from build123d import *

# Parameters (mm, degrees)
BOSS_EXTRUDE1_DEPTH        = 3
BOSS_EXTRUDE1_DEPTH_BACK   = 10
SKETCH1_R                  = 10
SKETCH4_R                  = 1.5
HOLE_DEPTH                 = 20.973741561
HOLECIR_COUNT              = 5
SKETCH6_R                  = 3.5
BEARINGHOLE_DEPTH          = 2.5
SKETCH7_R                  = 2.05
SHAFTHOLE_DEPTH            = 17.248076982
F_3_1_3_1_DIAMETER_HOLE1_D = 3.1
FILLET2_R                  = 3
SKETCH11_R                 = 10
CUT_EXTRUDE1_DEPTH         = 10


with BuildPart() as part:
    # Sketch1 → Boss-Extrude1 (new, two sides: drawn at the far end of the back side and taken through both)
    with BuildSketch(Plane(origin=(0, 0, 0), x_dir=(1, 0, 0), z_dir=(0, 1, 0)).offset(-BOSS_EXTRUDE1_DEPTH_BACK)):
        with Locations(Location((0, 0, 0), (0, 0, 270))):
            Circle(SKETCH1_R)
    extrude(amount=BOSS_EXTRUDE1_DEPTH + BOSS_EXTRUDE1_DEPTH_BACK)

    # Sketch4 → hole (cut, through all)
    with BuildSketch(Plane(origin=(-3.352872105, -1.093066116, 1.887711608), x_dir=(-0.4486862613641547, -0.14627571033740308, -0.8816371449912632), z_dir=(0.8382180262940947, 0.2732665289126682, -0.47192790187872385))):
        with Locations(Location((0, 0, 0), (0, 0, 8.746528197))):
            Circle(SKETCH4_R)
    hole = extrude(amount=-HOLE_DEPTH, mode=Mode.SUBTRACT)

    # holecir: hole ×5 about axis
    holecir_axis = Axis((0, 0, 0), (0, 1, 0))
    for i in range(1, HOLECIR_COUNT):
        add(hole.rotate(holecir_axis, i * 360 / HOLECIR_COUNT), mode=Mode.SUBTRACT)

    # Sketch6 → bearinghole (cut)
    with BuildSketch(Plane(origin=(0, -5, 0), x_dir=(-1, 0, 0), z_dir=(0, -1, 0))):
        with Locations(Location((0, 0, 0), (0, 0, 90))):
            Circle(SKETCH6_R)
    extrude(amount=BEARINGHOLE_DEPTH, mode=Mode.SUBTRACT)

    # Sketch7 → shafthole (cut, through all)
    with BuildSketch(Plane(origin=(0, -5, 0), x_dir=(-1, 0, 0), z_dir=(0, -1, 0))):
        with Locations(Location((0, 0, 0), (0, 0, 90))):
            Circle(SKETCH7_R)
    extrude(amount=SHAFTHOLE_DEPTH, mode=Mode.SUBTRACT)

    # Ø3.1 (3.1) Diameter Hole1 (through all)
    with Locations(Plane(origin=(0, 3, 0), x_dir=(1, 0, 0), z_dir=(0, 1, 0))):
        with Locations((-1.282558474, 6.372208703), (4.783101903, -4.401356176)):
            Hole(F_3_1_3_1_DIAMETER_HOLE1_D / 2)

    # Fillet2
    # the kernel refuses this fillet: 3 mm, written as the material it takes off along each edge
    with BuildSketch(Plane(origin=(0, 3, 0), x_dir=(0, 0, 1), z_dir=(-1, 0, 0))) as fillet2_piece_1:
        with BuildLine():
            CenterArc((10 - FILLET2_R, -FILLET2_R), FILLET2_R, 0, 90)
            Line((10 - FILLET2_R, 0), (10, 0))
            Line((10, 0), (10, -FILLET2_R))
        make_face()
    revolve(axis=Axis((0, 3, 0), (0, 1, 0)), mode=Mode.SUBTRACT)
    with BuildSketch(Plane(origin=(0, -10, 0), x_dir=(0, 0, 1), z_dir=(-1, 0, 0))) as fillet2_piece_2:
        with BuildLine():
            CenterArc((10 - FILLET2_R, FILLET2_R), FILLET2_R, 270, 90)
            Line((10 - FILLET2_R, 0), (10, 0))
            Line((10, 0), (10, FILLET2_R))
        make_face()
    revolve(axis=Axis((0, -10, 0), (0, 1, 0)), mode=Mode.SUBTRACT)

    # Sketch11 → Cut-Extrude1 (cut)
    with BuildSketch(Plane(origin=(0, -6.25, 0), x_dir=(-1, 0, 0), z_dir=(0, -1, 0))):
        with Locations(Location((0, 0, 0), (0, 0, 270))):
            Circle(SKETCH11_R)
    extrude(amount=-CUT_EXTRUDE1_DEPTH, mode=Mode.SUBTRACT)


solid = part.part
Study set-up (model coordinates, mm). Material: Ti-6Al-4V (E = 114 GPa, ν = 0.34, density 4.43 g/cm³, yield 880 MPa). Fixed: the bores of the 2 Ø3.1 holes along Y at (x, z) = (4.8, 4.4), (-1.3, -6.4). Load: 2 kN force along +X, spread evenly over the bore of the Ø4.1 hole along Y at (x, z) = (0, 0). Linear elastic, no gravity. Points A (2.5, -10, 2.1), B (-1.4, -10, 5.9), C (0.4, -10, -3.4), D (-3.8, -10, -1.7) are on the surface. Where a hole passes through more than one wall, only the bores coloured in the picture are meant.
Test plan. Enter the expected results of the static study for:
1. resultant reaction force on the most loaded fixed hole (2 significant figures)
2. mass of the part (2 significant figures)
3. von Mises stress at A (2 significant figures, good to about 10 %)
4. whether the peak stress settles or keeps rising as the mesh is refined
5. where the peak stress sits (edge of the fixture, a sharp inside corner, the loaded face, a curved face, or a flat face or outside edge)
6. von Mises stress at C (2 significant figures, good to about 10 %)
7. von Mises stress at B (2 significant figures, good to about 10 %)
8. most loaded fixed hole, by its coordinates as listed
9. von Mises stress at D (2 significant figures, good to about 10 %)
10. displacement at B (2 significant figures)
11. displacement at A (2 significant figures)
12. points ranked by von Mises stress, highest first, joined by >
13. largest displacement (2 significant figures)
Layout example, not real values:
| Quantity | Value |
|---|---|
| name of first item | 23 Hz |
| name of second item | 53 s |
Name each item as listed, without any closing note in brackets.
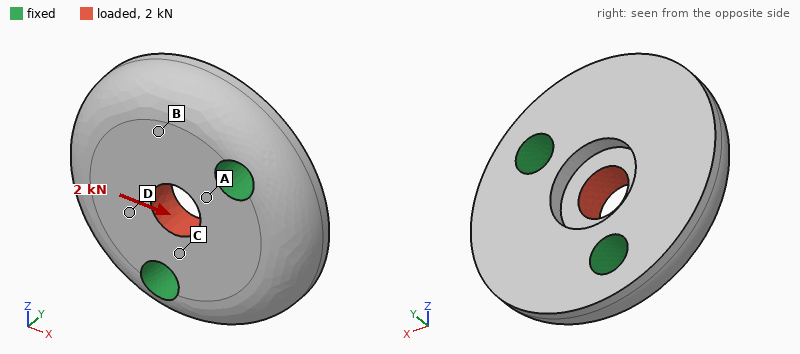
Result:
| Quantity | Value |
|---|---|
| resultant reaction force on the most loaded fixed hole | 1.1 kN |
| mass of the part | 4.1 g |
| von Mises stress at A | 67 MPa |
| whether the peak stress settles or keeps rising as the mesh is refined | keeps rising |
| where the peak stress sits | edge of the fixture |
| von Mises stress at C | 39 MPa |
| von Mises stress at B | 25 MPa |
| most loaded fixed hole, by its coordinates as listed | (4.8, 4.4) |
| von Mises stress at D | 49 MPa |
| displacement at B | 2.1 µm |
| displacement at A | 1.7 µm |
| points ranked by von Mises stress, highest first, joined by > | A > D > C > B |
| largest displacement | 4.5 µm |
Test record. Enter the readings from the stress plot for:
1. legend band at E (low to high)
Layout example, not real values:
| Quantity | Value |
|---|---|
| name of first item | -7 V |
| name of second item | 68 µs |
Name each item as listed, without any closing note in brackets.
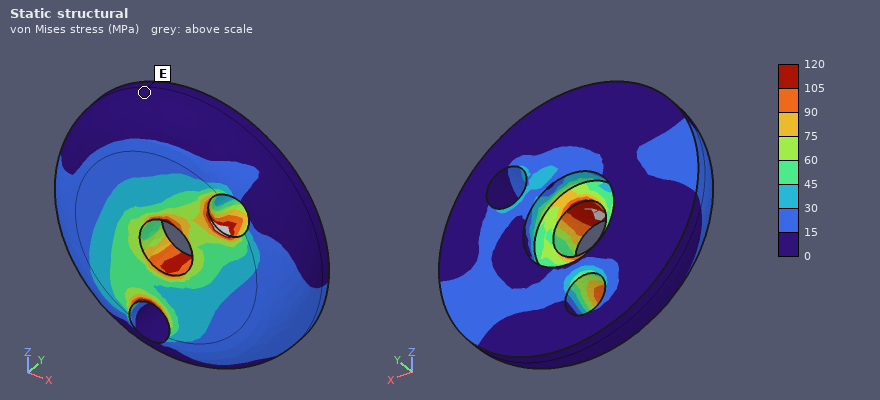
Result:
| Quantity | Value |
|---|---|
| legend band at E | 0 to 15 MPa |
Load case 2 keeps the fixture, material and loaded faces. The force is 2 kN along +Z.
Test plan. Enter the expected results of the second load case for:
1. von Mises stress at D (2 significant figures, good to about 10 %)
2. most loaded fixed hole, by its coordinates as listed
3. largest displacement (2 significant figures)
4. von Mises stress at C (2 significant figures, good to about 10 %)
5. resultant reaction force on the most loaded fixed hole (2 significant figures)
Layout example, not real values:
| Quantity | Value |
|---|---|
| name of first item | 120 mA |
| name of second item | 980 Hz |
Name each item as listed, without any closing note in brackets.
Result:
| Quantity | Value |
|---|---|
| von Mises stress at D | 26 MPa |
| most loaded fixed hole, by its coordinates as listed | (-1.3, -6.4) |
| largest displacement | 4.4 µm |
| von Mises stress at C | 64 MPa |
| resultant reaction force on the most loaded fixed hole | 1.1 kN |
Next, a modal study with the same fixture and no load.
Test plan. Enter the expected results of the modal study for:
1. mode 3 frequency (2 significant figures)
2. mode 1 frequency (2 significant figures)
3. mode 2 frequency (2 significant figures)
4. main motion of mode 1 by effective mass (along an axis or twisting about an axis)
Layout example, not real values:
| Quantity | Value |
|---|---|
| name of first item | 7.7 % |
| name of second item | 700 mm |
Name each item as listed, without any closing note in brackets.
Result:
| Quantity | Value |
|---|---|
| mode 3 frequency | 54 kHz |
| mode 1 frequency | 26 kHz |
| mode 2 frequency | 54 kHz |
| main motion of mode 1 by effective mass | along Y |
